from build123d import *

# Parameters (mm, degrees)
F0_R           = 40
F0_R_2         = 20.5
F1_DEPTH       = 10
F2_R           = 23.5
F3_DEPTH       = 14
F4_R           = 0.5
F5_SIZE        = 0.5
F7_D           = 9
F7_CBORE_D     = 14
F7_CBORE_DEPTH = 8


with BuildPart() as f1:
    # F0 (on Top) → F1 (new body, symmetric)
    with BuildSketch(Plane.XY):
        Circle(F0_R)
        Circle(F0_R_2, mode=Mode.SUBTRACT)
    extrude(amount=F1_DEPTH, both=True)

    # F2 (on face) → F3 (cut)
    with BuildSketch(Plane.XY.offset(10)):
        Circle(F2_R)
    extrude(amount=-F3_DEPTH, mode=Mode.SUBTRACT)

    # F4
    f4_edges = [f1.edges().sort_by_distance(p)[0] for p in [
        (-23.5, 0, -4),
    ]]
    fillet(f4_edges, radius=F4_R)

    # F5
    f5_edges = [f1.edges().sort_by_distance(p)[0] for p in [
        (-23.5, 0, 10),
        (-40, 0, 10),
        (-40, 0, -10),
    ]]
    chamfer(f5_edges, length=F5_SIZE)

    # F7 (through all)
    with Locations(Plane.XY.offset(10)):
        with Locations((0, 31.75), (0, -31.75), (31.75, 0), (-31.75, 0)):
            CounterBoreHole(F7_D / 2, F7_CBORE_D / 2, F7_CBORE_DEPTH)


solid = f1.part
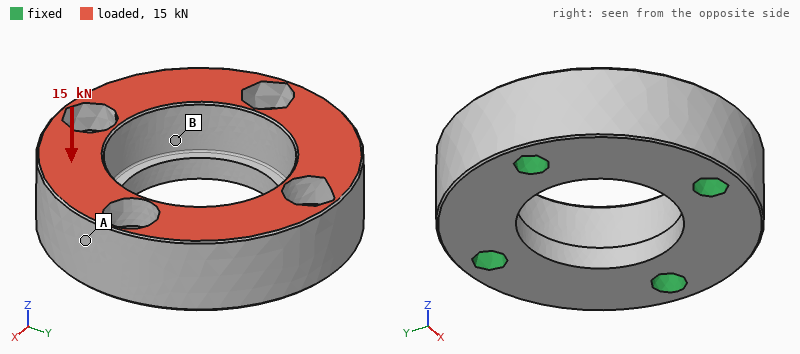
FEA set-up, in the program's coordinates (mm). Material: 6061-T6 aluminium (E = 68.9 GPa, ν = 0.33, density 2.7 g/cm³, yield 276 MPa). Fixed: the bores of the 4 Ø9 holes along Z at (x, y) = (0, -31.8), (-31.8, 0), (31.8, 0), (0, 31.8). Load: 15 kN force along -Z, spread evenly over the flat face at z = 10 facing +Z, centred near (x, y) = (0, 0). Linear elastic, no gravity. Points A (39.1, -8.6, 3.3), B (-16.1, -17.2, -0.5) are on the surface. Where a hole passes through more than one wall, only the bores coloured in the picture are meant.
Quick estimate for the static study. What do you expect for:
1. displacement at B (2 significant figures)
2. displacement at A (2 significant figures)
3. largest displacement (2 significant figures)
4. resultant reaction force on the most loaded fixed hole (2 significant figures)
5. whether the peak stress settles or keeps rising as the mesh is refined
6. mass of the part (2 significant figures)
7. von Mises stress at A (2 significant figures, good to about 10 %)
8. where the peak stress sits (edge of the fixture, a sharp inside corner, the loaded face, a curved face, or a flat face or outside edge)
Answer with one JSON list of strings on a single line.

["4.1 µm", "3.7 µm", "10 µm", "3.9 kN", "keeps rising", "160 g", "13 MPa", "edge of the fixture"]
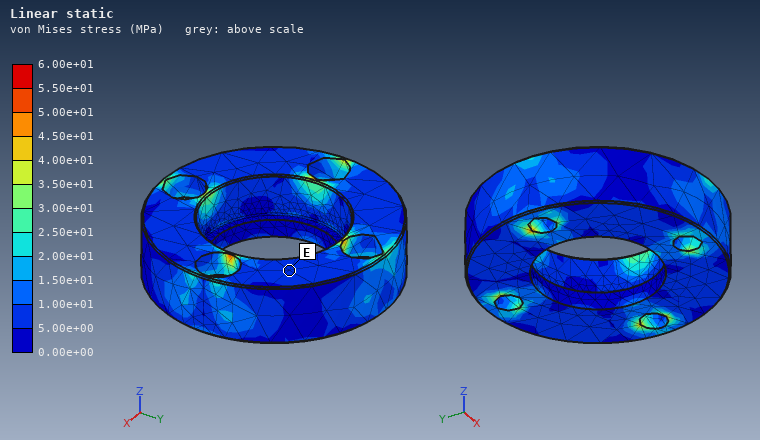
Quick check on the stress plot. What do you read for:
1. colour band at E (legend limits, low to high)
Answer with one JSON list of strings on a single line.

["5.00e+00 to 1.00e+01 MPa"]
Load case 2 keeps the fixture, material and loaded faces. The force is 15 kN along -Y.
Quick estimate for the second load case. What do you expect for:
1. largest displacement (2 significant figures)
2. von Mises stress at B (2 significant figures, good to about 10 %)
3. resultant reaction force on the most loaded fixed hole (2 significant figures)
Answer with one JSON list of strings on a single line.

["18 µm", "11 MPa", "5.1 kN"]
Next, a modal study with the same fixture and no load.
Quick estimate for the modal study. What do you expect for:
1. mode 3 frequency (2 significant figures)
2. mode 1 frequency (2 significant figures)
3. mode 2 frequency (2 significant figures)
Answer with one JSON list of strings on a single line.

["18 kHz", "16 kHz", "18 kHz"]
